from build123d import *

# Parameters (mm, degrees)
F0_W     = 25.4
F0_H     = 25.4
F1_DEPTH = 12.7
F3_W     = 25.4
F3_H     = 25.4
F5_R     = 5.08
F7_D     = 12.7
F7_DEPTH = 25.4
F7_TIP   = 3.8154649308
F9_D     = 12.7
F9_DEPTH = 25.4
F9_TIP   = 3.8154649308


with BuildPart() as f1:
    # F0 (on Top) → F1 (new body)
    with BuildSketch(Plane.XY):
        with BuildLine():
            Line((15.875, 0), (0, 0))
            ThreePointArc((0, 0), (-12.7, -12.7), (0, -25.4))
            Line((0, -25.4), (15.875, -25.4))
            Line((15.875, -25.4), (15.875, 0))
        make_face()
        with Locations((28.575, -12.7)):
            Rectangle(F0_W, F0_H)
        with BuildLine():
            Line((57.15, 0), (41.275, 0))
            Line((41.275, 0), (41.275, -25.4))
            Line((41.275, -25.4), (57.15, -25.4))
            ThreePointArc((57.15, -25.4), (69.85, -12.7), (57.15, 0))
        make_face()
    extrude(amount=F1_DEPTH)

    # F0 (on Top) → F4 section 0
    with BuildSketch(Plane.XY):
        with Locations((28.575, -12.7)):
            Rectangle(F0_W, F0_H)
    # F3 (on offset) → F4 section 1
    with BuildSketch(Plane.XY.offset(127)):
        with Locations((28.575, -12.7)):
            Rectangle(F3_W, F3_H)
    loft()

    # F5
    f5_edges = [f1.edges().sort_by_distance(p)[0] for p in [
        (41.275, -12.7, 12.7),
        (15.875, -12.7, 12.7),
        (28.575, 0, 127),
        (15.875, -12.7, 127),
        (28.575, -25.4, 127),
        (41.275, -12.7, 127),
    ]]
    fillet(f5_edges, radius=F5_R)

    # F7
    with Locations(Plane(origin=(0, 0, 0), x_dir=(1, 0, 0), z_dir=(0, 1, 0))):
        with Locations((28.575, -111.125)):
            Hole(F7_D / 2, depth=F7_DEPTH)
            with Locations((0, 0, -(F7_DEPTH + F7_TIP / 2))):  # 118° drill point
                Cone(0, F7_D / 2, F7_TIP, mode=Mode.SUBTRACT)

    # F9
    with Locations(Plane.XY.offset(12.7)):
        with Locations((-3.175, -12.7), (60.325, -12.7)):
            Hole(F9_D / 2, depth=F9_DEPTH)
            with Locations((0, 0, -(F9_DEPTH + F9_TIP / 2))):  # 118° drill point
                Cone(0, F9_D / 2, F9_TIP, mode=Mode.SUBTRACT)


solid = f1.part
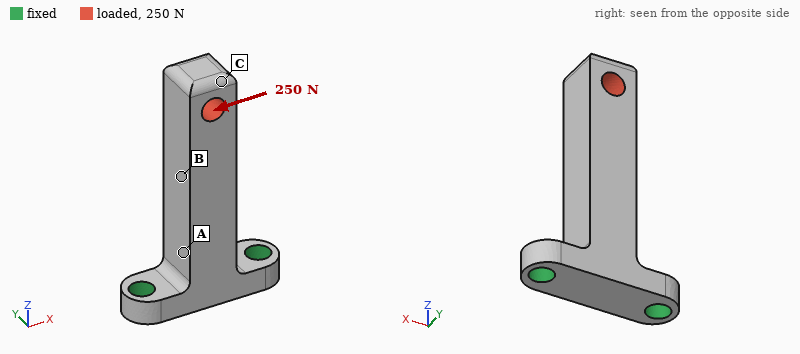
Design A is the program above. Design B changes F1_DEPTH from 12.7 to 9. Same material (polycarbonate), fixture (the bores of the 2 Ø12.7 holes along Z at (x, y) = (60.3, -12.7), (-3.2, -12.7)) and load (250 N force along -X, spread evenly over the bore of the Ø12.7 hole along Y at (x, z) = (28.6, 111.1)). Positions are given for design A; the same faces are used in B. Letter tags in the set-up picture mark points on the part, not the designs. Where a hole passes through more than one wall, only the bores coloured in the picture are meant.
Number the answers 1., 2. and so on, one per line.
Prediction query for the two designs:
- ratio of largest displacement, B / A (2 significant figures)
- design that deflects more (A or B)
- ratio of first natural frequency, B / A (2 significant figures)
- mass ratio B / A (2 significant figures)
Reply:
1. 1.3
2. B
3. 0.75
4. 0.96
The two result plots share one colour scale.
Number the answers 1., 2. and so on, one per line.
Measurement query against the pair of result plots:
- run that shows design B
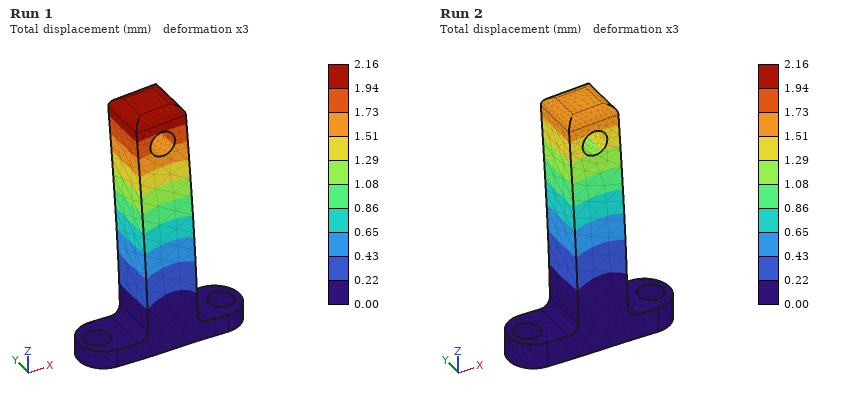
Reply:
1. Run 1
